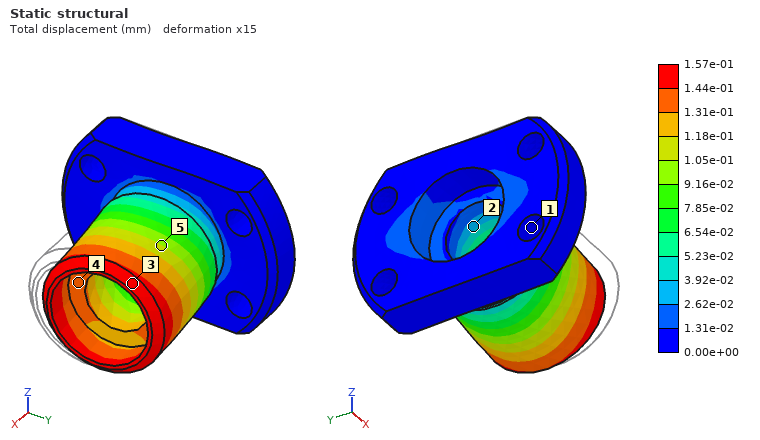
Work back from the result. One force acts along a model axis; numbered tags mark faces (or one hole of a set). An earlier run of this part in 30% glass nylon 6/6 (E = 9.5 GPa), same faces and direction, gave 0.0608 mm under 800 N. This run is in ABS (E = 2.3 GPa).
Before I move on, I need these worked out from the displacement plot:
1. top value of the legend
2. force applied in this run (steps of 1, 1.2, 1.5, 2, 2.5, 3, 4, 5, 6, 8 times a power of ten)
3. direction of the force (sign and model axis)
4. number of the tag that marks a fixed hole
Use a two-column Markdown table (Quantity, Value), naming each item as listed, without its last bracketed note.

| Quantity | Value |
|---|---|
| top value of the legend | 1.57e-01 mm |
| force applied in this run | 500 N |
| direction of the force | +Y |
| number of the tag that marks a fixed hole | 1 |
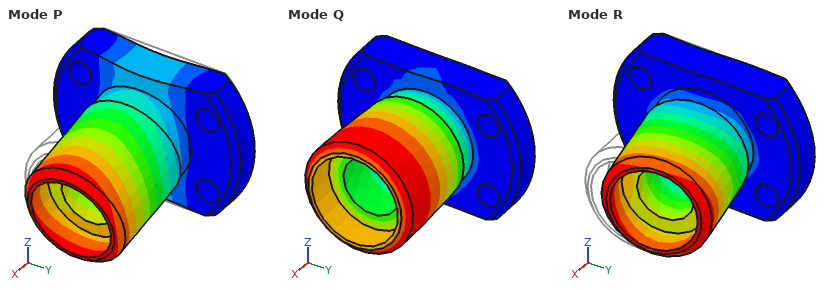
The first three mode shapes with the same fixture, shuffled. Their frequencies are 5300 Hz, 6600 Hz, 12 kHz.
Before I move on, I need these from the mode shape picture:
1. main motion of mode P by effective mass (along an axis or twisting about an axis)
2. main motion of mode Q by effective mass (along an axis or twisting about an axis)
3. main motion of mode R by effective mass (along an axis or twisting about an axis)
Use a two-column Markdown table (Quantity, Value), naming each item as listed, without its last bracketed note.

| Quantity | Value |
|---|---|
| main motion of mode P by effective mass | along Z |
| main motion of mode Q by effective mass | twisting about X |
| main motion of mode R by effective mass | along Y |
